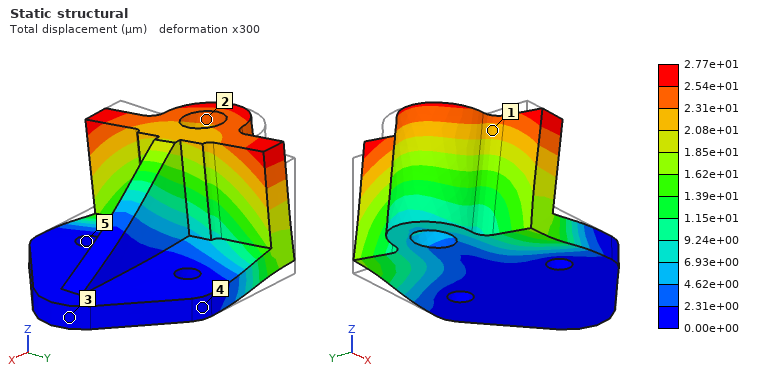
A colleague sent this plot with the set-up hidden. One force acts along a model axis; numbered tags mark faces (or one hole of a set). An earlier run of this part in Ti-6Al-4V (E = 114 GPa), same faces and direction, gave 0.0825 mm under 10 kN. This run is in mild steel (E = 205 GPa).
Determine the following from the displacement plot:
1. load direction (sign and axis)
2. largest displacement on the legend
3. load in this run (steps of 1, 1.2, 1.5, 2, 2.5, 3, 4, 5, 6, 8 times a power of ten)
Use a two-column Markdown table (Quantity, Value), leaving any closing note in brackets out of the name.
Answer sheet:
| Quantity | Value |
|---|---|
| load direction | -Y |
| largest displacement on the legend | 2.77e+01 µm |
| load in this run | 6 kN |
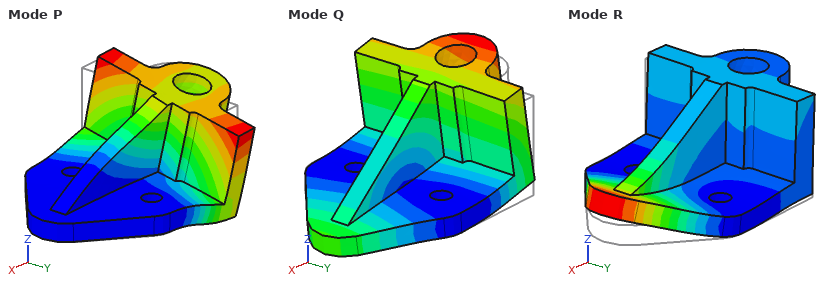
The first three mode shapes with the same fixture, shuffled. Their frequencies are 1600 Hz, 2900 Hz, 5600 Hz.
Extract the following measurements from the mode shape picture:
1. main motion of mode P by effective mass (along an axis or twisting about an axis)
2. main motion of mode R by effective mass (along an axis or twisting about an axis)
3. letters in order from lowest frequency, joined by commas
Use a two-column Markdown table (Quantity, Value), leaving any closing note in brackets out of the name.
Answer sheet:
| Quantity | Value |
|---|---|
| main motion of mode P by effective mass | along Y |
| main motion of mode R by effective mass | along Z |
| letters in order from lowest frequency, joined by commas | Q, P, R |
